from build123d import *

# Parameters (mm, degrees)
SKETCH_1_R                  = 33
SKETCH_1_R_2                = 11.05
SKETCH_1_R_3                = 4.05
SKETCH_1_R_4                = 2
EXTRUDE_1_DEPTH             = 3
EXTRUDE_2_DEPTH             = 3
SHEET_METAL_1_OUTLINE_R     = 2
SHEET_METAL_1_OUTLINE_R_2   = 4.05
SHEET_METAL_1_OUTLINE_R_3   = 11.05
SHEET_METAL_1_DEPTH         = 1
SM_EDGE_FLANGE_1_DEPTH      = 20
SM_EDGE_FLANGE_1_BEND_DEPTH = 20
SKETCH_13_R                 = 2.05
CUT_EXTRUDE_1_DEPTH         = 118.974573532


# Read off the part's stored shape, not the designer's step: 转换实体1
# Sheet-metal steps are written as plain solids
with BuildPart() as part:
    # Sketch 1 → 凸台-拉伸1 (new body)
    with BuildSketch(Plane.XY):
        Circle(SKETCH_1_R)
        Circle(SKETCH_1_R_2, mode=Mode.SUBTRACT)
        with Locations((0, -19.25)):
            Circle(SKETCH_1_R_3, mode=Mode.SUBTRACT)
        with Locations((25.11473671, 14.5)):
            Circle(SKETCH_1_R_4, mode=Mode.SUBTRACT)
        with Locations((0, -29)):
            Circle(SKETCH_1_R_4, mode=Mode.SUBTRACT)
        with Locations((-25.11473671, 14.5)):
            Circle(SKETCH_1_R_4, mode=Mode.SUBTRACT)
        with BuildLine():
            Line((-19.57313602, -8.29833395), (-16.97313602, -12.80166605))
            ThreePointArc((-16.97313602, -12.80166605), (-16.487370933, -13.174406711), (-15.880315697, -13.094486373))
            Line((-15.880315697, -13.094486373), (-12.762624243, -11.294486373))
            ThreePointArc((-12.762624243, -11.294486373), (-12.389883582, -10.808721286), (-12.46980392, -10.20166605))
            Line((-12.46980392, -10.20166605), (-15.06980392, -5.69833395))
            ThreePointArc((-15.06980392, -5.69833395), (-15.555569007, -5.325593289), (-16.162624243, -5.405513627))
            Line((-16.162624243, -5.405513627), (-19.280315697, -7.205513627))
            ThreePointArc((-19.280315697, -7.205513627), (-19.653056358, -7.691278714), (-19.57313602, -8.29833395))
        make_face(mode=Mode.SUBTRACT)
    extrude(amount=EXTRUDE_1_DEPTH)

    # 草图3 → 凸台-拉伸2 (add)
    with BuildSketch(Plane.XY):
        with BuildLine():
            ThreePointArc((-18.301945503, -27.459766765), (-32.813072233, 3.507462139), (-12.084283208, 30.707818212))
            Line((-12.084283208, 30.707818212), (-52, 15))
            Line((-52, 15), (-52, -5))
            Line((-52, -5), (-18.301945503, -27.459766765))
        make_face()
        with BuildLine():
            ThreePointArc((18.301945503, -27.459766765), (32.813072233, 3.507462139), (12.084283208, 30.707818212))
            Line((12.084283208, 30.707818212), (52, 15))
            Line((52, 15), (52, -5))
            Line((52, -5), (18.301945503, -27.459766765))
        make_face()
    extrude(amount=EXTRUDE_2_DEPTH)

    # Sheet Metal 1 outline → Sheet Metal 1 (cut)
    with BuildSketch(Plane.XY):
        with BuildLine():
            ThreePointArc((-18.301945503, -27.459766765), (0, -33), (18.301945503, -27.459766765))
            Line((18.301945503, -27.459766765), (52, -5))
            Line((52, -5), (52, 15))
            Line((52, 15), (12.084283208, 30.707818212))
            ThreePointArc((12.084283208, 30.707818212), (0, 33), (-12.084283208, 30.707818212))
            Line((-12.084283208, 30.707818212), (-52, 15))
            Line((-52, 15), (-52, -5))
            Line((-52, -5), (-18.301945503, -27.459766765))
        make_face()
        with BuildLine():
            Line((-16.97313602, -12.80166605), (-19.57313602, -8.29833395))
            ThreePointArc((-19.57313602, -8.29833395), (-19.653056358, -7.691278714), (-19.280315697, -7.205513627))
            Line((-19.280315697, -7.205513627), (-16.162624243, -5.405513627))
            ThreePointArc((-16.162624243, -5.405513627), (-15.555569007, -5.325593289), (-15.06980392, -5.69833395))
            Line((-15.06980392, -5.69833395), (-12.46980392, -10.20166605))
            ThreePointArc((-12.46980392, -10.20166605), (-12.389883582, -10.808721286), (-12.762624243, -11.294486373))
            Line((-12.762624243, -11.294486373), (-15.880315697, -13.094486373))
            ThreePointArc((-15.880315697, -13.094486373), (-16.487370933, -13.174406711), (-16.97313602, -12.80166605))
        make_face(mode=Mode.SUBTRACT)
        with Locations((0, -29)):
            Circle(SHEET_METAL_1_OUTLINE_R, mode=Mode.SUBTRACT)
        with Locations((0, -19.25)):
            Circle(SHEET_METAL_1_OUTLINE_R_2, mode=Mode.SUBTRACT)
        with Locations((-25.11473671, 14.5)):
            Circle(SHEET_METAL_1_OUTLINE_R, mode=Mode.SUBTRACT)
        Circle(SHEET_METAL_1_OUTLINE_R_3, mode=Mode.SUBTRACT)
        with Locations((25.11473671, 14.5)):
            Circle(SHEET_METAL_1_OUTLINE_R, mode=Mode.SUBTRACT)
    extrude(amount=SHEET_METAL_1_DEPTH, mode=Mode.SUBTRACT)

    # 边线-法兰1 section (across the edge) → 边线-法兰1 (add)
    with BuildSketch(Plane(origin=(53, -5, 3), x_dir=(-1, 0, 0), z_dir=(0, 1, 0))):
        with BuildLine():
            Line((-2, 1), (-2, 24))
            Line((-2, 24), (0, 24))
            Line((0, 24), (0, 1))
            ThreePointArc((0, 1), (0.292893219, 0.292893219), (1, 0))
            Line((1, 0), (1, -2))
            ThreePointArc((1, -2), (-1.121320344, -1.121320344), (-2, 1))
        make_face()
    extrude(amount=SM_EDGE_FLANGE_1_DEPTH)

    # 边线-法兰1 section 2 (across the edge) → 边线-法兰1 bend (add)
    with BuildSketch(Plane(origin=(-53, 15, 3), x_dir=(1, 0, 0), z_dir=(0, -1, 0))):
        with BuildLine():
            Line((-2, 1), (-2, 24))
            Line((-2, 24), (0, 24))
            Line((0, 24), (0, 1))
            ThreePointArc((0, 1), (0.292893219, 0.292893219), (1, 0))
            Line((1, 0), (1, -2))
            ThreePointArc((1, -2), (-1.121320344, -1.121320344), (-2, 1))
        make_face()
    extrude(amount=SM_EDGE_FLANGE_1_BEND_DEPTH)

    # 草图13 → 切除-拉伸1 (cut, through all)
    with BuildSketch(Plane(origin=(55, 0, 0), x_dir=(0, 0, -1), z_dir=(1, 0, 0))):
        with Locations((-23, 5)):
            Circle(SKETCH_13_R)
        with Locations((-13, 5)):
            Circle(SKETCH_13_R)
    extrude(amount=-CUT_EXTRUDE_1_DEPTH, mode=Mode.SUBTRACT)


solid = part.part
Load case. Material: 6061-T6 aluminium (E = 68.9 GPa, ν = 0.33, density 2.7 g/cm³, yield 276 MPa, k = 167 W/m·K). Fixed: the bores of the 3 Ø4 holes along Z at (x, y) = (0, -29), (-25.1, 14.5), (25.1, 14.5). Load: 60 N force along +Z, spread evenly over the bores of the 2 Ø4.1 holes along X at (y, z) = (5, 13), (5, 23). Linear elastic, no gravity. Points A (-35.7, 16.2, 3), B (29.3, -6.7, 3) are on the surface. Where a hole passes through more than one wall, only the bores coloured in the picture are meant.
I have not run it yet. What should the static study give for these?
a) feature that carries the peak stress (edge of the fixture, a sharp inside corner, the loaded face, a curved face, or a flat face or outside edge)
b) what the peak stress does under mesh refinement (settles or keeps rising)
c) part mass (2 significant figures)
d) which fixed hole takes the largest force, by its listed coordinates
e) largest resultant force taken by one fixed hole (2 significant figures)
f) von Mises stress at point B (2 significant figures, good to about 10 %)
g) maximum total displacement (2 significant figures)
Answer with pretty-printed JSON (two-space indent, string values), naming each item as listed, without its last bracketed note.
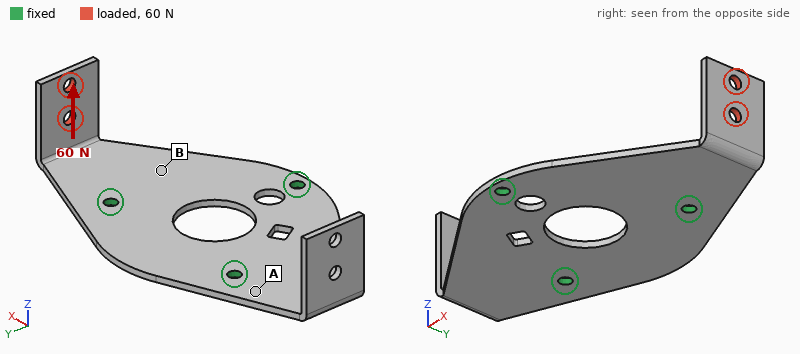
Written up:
{
  "feature that carries the peak stress": "edge of the fixture",
  "what the peak stress does under mesh refinement": "keeps rising",
  "part mass": "29 g",
  "which fixed hole takes the largest force, by its listed coordinates": "(25.1, 14.5)",
  "largest resultant force taken by one fixed hole": "70 N",
  "von Mises stress at point B": "32 MPa",
  "maximum total displacement": "0.62 mm"
}
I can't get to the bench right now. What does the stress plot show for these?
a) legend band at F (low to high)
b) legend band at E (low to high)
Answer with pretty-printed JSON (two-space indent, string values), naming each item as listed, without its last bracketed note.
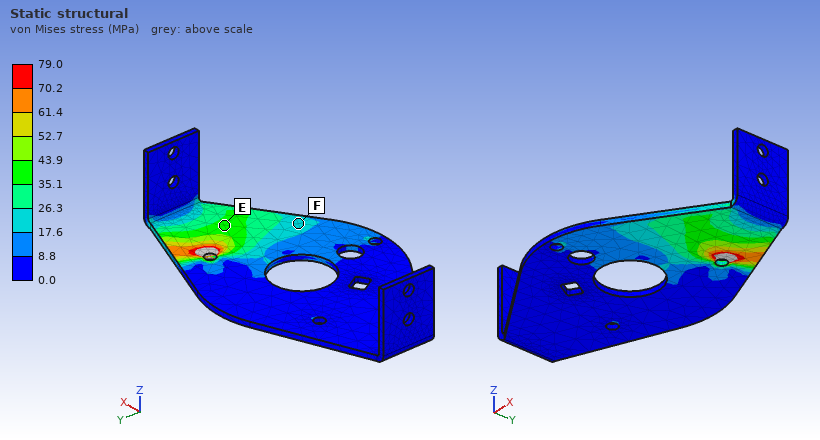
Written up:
{
  "legend band at F": "17.6 to 26.3 MPa",
  "legend band at E": "35.1 to 43.9 MPa"
}
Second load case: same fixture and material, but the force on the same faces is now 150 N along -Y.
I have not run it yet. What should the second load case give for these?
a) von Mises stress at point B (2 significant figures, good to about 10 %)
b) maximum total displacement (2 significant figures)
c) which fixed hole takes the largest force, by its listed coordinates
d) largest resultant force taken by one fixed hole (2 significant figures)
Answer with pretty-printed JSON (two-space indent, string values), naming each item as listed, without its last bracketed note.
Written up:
{
  "von Mises stress at point B": "49 MPa",
  "maximum total displacement": "0.95 mm",
  "which fixed hole takes the largest force, by its listed coordinates": "(25.1, 14.5)",
  "largest resultant force taken by one fixed hole": "160 N"
}
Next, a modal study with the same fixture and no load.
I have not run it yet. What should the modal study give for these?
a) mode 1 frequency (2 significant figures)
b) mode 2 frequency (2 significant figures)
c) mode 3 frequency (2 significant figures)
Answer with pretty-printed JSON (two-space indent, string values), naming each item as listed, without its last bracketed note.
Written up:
{
  "mode 1 frequency": "890 Hz",
  "mode 2 frequency": "900 Hz",
  "mode 3 frequency": "1600 Hz"
}
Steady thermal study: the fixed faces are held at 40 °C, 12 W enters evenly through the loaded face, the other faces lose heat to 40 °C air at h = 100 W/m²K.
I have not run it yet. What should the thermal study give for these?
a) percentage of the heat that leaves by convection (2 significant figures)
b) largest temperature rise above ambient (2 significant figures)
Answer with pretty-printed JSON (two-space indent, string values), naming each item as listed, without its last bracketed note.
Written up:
{
  "percentage of the heat that leaves by convection": "55 %",
  "largest temperature rise above ambient": "49 K"
}
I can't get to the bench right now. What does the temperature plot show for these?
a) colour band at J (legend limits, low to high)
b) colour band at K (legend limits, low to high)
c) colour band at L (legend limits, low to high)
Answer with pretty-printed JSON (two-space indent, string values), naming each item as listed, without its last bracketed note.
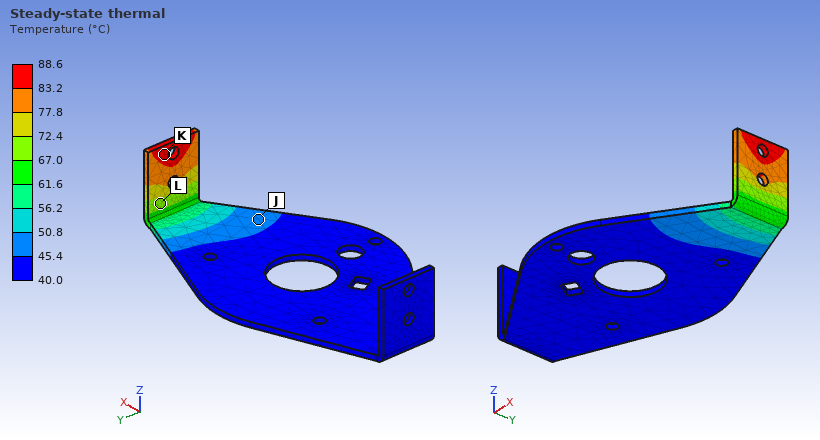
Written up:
{
  "colour band at J": "45.4 to 50.8 °C",
  "colour band at K": "83.2 to 88.6 °C",
  "colour band at L": "67.0 to 72.4 °C"
}
